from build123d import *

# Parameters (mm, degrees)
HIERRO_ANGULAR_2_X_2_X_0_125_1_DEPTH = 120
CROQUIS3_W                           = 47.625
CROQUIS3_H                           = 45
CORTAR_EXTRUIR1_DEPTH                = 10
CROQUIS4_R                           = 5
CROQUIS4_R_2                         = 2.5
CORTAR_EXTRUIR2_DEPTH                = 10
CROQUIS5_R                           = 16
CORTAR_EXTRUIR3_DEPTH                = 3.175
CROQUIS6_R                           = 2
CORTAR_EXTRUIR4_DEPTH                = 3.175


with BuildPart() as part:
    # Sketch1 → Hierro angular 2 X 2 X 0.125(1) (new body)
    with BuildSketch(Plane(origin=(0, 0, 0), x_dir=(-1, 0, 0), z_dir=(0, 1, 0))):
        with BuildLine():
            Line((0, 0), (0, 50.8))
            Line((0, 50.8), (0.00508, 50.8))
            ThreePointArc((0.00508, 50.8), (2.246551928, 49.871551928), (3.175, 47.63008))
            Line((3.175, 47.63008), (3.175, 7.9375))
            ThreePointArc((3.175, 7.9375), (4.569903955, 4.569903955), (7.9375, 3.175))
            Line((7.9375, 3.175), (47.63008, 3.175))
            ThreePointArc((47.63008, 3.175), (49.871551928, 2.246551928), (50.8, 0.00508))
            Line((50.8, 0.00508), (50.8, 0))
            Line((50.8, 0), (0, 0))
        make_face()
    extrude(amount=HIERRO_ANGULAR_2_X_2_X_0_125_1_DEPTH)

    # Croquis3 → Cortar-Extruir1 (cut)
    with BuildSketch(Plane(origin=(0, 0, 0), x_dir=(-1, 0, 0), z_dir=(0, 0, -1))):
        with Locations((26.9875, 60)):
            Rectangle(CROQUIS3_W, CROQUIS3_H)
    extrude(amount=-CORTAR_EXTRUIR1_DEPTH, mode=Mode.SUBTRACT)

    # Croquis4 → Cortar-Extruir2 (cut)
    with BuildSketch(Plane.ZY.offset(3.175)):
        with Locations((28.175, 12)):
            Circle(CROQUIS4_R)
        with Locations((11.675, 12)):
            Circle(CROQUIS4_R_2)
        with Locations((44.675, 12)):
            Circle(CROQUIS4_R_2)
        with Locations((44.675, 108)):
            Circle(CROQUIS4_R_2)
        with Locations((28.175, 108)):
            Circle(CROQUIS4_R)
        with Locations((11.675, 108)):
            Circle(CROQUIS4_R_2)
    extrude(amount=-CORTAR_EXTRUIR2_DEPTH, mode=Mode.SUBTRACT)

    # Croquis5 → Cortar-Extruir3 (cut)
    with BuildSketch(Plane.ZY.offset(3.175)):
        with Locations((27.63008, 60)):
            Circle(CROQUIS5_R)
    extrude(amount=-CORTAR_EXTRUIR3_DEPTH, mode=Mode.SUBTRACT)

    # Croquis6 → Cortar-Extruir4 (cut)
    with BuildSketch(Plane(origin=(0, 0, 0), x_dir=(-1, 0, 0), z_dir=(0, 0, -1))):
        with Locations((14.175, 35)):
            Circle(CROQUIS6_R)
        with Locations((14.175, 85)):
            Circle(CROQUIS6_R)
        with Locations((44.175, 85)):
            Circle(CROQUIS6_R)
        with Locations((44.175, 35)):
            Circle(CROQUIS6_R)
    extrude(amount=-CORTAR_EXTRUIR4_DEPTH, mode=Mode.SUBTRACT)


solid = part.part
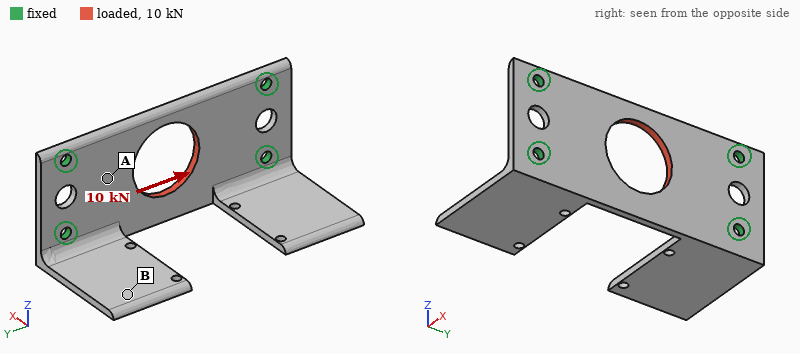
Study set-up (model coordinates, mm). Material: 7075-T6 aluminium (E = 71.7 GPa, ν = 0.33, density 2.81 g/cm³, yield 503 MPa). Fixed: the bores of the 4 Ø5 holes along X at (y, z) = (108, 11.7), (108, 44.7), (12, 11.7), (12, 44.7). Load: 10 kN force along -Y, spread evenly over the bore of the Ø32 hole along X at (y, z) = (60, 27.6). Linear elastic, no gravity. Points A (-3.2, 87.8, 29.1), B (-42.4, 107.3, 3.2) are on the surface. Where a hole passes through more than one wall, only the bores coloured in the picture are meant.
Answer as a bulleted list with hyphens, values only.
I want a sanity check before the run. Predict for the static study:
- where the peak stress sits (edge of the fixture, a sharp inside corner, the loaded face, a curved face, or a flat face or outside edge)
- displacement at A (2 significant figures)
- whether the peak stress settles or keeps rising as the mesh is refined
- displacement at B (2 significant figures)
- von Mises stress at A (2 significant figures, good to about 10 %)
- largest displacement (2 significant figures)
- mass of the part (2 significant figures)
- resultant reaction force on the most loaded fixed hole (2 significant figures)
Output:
- edge of the fixture
- 13 µm
- keeps rising
- 9.4 µm
- 27 MPa
- 27 µm
- 76 g
- 2.8 kN
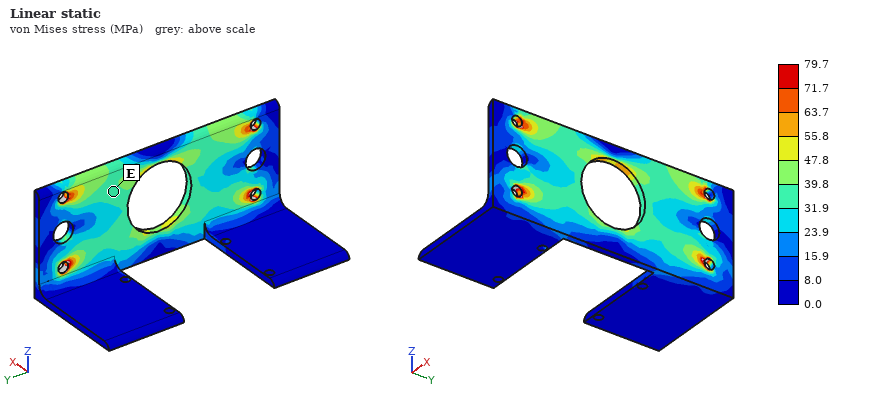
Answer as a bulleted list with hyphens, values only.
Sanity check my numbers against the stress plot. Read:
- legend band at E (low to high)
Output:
- 31.9 to 39.8 MPa
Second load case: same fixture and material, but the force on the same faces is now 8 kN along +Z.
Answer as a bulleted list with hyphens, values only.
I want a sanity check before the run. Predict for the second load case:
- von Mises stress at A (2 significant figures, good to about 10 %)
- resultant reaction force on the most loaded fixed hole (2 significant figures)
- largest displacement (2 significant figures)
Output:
- 77 MPa
- 3.1 kN
- 90 µm
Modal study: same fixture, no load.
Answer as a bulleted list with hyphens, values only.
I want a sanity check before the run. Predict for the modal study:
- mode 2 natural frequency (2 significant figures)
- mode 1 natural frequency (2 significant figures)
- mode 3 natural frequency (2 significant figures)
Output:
- 970 Hz
- 940 Hz
- 1500 Hz
